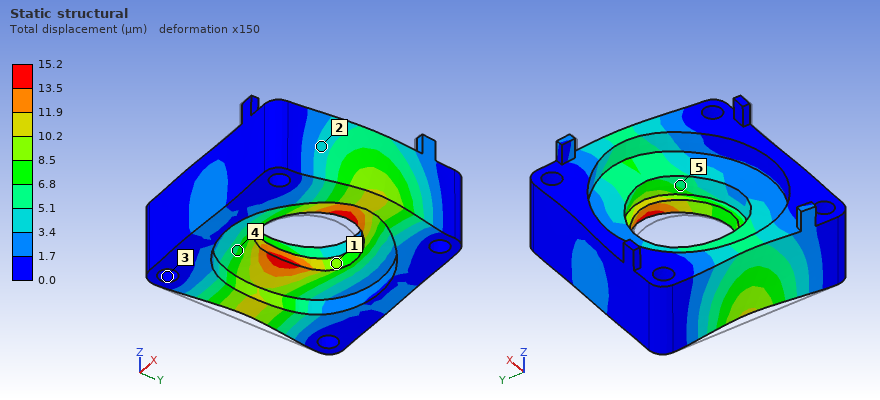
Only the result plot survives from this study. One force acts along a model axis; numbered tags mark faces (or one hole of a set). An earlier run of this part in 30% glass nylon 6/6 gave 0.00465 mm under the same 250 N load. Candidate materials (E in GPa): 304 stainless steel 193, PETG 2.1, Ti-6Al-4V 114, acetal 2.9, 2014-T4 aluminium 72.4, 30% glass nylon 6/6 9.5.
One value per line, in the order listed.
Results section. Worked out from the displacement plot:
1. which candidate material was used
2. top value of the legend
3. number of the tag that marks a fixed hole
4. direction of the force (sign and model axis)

acetal
15.2 µm
3
+X
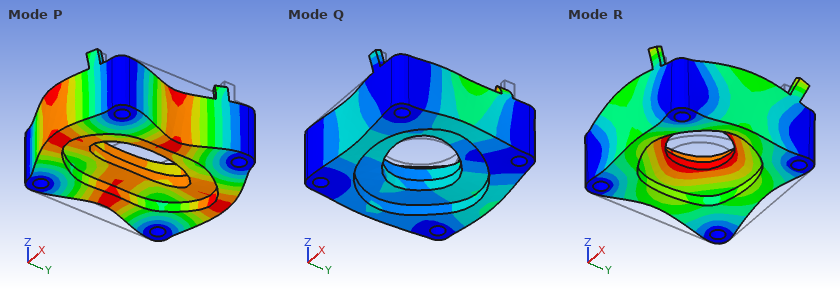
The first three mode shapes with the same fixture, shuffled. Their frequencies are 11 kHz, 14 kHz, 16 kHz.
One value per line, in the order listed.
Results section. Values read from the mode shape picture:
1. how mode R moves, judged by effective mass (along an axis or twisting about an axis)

along Z
